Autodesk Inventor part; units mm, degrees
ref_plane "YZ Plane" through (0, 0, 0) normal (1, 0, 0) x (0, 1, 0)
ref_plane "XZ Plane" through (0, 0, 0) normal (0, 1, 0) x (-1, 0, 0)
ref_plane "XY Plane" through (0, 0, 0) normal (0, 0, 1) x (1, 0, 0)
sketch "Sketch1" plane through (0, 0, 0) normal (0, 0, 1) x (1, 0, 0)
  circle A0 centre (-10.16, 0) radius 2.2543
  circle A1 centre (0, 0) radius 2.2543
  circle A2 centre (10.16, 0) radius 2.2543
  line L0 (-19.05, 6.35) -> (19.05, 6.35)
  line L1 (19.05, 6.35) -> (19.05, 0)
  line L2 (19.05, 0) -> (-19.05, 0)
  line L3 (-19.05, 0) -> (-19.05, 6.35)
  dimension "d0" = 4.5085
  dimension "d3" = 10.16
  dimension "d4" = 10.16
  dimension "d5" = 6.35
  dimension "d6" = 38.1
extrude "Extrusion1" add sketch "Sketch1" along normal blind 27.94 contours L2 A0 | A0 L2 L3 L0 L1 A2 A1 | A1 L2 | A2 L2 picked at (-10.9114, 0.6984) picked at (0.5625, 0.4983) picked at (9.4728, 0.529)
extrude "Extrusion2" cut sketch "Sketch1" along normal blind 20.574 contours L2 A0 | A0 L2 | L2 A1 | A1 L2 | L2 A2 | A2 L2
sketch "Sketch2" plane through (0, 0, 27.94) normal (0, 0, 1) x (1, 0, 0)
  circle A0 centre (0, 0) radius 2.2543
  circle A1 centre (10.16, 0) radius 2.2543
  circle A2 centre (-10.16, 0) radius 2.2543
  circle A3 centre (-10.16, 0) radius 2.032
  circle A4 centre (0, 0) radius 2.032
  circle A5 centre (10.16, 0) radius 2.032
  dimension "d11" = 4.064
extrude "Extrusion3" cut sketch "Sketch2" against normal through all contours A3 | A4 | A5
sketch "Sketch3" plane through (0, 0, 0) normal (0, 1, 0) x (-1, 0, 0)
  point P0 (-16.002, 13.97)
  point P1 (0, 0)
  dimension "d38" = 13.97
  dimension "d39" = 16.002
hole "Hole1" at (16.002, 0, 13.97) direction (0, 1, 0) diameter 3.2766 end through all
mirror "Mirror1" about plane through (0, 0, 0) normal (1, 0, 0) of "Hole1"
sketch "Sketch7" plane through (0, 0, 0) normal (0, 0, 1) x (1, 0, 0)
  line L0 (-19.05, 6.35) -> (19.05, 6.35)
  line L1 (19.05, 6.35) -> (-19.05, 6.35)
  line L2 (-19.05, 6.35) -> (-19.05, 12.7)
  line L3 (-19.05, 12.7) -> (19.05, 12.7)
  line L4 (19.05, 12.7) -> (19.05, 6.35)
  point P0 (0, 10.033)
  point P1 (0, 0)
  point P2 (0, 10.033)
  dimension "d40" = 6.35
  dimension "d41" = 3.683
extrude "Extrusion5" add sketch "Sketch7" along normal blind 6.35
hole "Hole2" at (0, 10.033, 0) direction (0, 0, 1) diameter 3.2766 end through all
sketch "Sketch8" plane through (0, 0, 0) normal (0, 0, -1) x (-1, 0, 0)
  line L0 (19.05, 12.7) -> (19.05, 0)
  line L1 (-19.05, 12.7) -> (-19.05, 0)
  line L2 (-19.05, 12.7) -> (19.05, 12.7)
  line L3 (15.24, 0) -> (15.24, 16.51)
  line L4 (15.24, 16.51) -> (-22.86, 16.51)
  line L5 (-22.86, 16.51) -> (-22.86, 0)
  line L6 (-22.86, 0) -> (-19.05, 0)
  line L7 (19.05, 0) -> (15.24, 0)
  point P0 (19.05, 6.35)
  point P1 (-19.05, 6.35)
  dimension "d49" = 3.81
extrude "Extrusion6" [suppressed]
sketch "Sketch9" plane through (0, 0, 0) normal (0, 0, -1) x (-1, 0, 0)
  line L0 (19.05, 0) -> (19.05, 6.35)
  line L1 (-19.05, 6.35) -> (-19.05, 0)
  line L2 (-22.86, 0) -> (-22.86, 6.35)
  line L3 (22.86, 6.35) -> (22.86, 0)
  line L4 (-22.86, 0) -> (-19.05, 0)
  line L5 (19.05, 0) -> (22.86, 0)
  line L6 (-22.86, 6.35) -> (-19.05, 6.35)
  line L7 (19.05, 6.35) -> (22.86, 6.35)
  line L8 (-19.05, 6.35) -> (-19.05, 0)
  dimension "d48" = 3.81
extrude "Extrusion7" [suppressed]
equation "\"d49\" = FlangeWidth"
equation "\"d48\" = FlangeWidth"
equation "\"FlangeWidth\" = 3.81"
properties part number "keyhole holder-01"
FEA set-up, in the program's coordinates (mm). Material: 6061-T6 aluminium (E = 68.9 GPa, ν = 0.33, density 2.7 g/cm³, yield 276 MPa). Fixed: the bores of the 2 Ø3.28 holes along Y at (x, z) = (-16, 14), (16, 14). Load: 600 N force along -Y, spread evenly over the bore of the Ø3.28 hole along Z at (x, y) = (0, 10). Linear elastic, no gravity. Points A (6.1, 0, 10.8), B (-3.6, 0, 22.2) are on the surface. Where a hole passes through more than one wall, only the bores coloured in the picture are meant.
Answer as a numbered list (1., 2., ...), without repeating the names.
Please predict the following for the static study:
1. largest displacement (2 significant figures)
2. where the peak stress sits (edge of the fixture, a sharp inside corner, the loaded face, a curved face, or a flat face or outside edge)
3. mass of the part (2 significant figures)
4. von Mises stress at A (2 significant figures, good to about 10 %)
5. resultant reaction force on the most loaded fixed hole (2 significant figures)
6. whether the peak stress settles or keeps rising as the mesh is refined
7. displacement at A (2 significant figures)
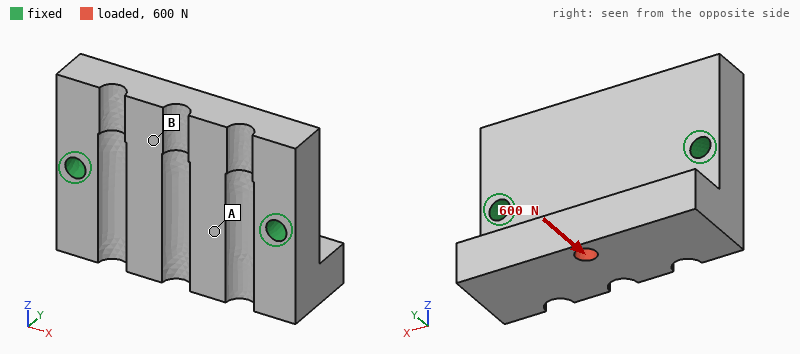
1. 23 µm
2. edge of the fixture
3. 20 g
4. 12 MPa
5. 310 N
6. keeps rising
7. 6.0 µm
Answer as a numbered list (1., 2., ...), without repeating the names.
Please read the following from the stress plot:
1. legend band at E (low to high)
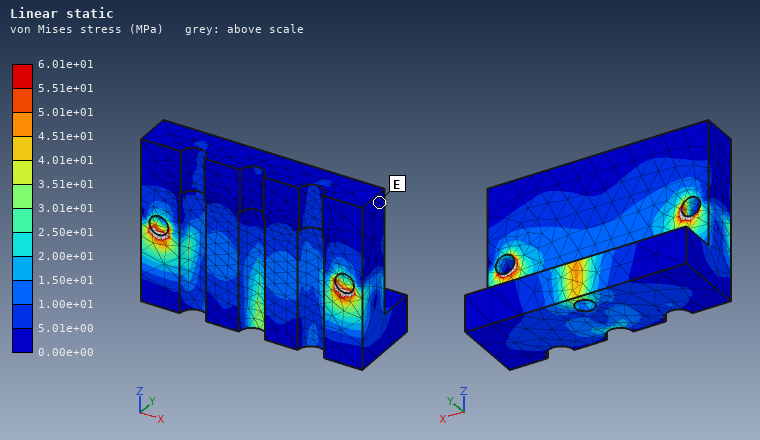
1. 0.00e+00 to 5.01e+00 MPa
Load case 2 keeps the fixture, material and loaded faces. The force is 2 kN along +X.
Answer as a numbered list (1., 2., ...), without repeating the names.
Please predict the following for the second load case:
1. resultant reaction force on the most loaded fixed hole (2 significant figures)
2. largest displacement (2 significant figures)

1. 1.3 kN
2. 15 µm
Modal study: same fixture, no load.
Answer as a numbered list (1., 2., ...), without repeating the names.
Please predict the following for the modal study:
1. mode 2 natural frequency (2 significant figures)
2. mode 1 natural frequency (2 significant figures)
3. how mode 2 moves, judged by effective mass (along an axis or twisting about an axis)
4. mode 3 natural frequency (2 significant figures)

1. 16 kHz
2. 11 kHz
3. along Y
4. 20 kHz
